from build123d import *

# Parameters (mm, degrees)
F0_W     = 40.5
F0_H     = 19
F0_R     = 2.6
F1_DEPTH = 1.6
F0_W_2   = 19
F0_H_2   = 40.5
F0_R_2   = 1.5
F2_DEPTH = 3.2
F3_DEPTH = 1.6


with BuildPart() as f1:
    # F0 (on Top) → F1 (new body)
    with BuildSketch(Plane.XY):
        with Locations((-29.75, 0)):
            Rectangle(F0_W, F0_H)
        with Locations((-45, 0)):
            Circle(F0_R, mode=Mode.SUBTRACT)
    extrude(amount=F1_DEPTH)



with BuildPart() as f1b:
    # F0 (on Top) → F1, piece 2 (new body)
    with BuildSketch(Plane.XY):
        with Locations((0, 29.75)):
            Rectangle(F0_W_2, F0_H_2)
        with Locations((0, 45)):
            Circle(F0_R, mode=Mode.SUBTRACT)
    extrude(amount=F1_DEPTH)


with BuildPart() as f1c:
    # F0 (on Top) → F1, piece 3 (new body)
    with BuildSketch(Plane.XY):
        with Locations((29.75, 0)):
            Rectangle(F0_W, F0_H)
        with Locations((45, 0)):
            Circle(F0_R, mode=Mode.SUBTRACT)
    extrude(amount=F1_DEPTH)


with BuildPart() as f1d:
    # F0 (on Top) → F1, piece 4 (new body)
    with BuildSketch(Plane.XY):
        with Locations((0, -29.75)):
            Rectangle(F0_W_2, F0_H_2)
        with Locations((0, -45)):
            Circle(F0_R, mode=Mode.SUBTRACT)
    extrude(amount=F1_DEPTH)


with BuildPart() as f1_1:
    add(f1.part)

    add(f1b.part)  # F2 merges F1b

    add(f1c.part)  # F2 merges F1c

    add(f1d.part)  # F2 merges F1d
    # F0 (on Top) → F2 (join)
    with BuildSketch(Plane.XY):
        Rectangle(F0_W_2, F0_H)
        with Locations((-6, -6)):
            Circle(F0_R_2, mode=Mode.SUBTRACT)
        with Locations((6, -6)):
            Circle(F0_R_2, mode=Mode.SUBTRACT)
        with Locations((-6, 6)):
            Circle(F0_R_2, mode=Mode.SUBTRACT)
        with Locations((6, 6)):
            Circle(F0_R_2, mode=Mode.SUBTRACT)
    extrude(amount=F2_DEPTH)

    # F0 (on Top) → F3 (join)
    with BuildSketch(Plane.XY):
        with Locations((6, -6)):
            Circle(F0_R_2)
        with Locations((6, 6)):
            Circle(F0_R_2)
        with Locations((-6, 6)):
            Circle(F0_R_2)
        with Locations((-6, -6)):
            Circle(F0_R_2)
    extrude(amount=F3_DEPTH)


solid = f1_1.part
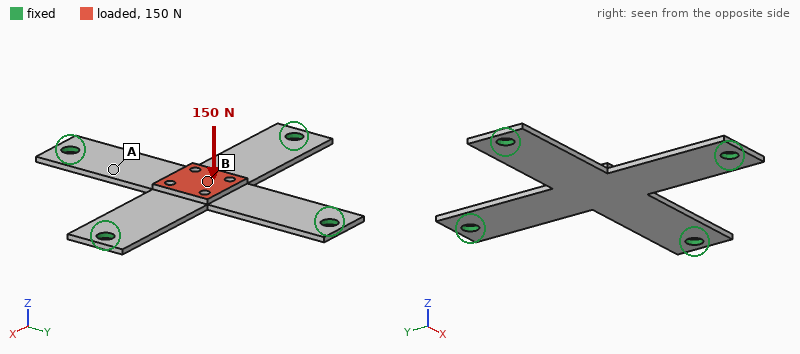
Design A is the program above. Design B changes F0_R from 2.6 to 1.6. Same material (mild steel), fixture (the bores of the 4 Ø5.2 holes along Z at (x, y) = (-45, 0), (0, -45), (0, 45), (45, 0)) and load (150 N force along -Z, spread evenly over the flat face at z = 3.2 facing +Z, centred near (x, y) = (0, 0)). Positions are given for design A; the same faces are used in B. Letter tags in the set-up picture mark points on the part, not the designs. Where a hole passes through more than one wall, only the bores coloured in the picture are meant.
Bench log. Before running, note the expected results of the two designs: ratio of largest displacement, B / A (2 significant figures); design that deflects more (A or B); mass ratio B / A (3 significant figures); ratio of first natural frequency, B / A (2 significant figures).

1.1
B
1.01
0.93
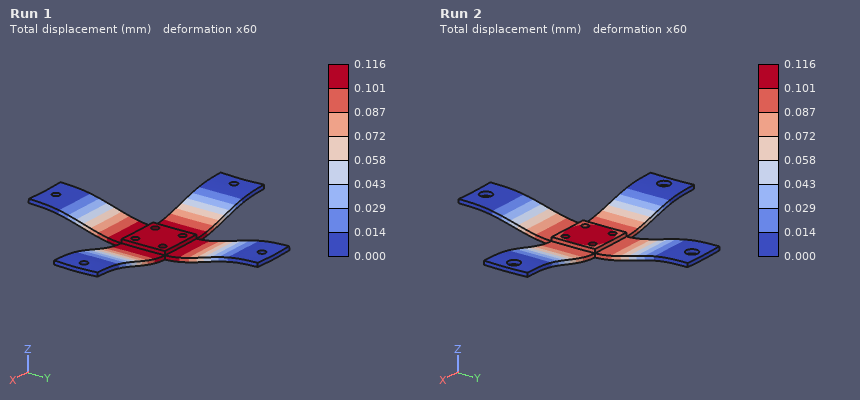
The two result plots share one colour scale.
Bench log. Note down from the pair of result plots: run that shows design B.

Run 1
